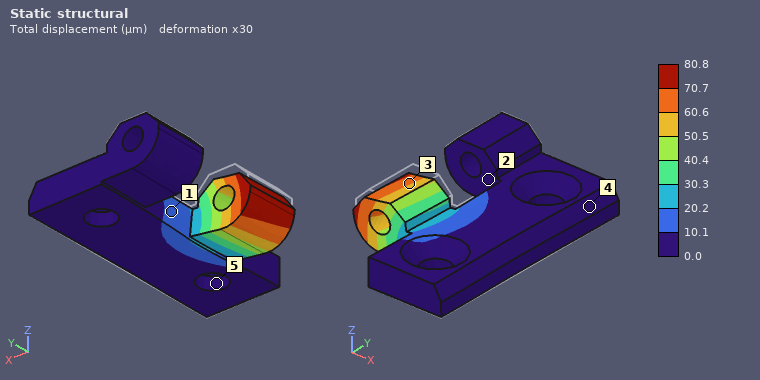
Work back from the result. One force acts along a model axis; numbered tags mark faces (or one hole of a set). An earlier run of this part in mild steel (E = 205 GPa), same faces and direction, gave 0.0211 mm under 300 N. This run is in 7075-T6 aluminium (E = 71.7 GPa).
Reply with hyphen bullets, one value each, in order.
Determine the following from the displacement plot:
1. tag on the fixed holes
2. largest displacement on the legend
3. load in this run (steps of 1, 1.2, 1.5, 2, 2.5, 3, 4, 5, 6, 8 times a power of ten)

- 5
- 80.8 µm
- 400 N
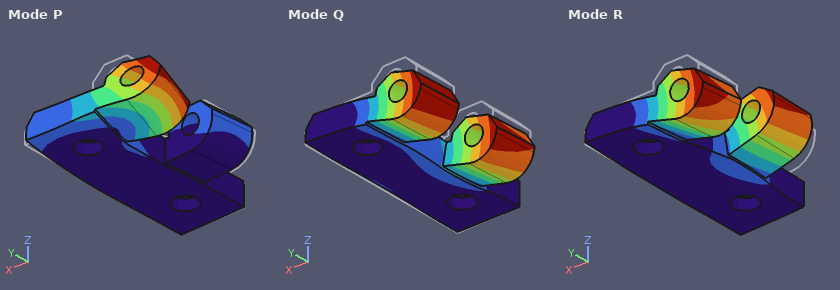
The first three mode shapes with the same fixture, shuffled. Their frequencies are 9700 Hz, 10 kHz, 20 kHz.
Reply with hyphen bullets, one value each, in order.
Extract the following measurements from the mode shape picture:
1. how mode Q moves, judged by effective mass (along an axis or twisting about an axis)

- along Z
